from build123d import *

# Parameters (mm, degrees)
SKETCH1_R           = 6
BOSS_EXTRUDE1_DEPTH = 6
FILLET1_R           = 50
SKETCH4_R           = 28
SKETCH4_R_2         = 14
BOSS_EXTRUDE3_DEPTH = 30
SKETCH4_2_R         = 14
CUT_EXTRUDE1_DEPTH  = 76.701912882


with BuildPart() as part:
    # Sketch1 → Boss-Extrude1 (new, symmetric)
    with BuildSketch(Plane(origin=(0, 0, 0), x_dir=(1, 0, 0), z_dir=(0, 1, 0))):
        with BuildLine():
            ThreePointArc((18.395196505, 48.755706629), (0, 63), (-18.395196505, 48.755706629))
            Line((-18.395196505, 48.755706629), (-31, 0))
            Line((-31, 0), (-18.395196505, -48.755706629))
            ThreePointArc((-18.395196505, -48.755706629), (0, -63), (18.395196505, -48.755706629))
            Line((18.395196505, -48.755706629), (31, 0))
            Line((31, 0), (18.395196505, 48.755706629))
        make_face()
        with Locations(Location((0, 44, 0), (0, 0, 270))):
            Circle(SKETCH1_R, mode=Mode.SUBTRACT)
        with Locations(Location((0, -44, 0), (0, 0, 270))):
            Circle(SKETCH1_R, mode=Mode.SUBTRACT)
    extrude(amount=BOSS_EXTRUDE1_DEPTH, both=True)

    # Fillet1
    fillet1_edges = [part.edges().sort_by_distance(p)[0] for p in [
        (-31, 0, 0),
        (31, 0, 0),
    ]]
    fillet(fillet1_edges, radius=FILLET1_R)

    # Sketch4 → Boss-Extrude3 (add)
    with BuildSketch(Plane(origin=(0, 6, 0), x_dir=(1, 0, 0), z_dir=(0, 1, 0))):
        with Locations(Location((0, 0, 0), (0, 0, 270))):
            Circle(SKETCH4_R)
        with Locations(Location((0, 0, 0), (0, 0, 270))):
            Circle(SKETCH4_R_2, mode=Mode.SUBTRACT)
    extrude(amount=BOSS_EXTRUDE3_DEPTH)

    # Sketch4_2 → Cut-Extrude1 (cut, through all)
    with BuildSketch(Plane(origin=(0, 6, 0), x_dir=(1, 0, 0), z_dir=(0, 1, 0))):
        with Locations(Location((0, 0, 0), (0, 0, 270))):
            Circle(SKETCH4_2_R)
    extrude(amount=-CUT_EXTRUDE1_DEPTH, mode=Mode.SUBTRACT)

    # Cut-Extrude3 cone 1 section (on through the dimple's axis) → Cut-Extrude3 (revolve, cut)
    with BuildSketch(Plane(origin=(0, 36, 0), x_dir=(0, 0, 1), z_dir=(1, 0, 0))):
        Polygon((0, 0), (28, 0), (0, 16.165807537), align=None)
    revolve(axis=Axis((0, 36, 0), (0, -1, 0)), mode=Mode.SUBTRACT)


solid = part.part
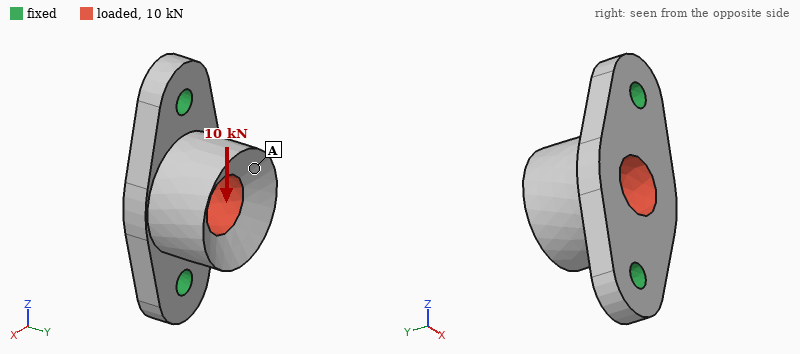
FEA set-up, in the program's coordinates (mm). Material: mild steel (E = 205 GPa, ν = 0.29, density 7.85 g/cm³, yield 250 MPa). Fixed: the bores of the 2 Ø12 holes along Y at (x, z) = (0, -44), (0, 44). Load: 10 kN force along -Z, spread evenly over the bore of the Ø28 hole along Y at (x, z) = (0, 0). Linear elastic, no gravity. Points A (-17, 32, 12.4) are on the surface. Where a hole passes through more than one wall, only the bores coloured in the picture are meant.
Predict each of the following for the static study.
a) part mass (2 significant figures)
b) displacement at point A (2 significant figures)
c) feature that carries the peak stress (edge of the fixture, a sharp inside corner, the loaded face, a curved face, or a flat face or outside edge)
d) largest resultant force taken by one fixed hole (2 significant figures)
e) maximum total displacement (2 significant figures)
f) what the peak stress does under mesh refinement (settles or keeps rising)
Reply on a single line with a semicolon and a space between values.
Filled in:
830 g; 3.7 µm; edge of the fixture; 5.2 kN; 4.3 µm; keeps rising
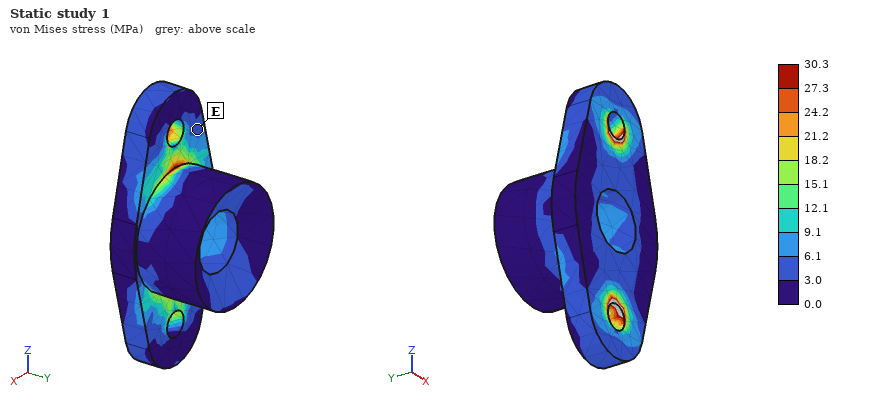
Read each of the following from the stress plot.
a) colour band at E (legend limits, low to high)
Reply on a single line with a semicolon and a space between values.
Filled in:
3.0 to 6.1 MPa
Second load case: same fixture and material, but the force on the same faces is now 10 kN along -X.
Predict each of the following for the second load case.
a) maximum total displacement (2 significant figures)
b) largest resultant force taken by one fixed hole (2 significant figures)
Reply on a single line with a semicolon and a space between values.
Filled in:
29 µm; 5.0 kN
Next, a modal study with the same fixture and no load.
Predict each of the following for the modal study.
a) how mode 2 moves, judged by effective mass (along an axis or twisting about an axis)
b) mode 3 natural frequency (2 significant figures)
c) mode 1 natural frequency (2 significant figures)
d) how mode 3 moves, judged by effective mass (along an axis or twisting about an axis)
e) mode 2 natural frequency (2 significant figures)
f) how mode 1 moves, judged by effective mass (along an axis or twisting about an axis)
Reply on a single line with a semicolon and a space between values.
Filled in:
along Y; 10 kHz; 3800 Hz; along Z; 6900 Hz; along X
